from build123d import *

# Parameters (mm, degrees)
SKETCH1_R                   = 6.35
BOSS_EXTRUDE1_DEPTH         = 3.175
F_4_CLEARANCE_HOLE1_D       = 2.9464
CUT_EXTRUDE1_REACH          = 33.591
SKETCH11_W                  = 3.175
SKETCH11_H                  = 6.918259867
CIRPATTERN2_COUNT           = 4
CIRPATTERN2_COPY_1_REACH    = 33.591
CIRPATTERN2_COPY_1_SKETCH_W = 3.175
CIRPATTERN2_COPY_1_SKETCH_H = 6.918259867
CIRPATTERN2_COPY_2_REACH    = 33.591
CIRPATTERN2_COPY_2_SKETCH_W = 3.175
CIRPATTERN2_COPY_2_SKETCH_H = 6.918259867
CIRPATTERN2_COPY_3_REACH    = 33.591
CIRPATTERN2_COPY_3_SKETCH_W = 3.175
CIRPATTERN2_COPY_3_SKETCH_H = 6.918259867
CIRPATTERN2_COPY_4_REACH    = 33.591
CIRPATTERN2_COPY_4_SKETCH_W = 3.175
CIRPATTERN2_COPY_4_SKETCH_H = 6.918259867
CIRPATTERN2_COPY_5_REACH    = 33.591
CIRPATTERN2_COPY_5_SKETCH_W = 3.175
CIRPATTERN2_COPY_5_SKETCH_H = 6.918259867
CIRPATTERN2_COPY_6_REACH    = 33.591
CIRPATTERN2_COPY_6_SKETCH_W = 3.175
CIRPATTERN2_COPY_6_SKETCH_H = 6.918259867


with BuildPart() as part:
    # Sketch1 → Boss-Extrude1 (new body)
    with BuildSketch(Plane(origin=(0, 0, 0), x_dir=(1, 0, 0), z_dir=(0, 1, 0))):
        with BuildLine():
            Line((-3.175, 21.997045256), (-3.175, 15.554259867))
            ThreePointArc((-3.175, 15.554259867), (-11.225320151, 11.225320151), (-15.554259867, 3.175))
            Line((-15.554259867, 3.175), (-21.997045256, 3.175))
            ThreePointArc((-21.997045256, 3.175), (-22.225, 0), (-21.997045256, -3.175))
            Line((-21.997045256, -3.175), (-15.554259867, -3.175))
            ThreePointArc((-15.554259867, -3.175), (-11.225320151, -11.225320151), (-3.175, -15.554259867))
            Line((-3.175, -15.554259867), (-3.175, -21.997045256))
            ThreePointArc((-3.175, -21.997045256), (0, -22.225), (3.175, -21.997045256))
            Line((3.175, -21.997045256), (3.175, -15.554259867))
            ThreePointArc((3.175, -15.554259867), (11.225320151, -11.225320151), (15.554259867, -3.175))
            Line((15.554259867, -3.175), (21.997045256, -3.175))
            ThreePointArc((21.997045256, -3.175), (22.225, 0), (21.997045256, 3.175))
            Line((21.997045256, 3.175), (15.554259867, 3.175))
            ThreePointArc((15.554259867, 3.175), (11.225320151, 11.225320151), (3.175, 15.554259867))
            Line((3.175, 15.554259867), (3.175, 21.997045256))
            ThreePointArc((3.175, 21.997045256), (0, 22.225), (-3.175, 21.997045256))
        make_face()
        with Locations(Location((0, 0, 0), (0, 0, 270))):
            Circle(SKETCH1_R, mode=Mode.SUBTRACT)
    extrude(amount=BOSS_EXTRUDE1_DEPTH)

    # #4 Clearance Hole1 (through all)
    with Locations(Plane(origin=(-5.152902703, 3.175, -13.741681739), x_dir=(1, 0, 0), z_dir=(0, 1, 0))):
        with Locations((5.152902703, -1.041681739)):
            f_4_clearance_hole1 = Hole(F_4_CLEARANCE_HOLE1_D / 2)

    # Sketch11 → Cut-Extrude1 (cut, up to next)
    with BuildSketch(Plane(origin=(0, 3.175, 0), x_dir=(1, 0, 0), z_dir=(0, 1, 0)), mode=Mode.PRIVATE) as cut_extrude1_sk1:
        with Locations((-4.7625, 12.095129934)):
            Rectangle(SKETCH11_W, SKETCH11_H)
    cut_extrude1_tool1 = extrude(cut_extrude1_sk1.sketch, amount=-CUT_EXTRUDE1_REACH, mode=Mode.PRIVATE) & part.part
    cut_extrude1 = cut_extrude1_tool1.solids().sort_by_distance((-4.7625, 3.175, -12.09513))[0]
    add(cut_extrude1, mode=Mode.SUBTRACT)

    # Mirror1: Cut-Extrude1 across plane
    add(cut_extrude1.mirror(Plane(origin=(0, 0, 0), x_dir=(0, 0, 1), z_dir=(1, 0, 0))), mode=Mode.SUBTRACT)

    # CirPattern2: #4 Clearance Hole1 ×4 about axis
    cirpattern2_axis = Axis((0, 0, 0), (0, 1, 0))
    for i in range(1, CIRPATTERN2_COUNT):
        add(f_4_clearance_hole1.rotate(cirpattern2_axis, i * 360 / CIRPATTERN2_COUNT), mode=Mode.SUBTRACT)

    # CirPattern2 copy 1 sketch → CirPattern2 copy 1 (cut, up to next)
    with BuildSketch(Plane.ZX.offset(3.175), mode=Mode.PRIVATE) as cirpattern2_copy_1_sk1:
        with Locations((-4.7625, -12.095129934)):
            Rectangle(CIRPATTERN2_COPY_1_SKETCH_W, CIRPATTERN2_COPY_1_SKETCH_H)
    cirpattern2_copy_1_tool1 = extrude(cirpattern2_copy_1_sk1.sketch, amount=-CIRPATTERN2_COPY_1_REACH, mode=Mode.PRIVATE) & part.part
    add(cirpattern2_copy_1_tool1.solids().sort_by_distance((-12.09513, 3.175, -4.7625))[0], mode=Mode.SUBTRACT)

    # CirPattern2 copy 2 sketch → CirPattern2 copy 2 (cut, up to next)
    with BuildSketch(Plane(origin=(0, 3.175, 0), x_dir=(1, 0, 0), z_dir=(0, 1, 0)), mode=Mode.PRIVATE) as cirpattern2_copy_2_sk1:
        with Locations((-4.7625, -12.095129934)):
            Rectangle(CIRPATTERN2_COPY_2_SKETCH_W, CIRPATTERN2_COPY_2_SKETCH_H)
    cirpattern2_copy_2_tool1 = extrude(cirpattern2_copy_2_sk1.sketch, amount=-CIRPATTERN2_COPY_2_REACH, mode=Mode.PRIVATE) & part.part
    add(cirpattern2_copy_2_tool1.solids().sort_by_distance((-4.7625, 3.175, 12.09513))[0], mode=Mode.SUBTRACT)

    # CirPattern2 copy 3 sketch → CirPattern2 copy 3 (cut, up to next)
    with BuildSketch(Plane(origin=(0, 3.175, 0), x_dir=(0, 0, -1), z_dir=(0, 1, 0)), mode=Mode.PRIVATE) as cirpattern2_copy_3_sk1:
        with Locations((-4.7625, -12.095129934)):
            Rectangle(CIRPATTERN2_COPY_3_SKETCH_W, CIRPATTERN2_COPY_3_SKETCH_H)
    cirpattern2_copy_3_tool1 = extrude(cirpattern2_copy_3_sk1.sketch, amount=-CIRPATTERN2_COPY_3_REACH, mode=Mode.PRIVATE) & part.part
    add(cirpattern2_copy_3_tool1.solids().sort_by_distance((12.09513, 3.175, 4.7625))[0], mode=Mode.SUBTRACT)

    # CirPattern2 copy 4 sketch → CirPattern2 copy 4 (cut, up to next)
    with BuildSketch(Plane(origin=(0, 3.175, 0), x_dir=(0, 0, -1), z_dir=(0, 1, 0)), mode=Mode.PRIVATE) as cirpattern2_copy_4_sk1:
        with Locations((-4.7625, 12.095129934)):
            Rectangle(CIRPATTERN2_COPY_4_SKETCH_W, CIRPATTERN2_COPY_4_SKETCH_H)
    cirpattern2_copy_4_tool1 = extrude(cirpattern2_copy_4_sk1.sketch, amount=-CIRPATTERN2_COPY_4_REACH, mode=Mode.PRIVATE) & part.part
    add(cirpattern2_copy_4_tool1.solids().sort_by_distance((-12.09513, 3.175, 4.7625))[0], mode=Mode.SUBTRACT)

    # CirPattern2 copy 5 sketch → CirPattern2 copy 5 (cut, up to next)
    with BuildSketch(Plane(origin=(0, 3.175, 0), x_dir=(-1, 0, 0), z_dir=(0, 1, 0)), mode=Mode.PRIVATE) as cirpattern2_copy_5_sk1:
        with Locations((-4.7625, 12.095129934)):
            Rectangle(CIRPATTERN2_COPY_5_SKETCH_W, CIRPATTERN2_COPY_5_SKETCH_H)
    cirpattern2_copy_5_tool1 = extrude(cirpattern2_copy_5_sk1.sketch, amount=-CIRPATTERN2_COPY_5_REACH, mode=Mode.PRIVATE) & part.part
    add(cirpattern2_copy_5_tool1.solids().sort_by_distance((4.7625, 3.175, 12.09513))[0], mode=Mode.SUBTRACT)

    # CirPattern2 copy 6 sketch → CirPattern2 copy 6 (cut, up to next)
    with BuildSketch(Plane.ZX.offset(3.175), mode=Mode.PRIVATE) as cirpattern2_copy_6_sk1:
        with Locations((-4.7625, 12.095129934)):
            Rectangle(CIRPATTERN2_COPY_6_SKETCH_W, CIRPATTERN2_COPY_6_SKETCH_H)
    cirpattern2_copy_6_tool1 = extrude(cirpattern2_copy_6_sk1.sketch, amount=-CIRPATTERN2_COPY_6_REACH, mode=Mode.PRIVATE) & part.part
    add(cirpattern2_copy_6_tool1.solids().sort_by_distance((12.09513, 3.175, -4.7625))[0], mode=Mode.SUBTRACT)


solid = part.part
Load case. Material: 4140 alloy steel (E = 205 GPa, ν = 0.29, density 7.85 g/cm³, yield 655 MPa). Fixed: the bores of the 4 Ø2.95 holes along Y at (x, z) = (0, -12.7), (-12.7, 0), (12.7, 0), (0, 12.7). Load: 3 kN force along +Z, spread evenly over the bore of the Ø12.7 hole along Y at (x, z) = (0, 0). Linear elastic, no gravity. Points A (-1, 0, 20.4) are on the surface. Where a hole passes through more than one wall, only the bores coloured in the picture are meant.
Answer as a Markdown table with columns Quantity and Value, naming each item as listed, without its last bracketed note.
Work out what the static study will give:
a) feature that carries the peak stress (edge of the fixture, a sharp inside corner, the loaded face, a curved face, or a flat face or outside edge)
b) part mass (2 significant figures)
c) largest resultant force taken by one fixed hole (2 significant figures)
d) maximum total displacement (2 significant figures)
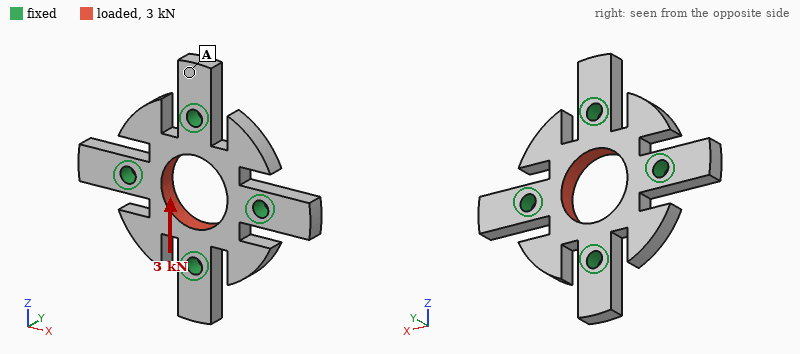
| Quantity | Value |
|---|---|
| feature that carries the peak stress | edge of the fixture |
| part mass | 16 g |
| largest resultant force taken by one fixed hole | 970 N |
| maximum total displacement | 5.3 µm |
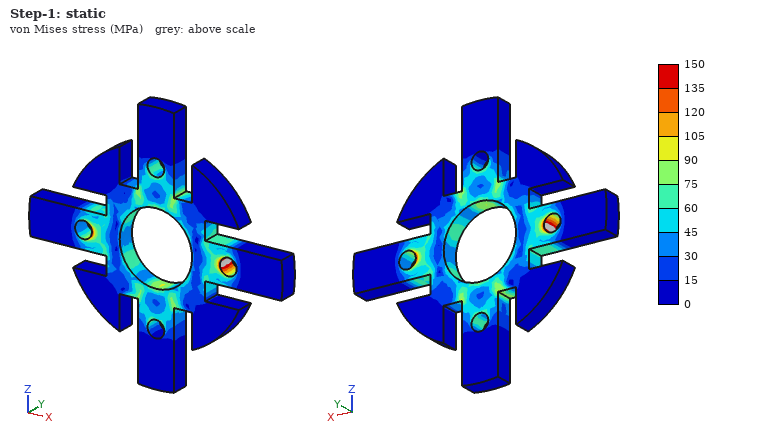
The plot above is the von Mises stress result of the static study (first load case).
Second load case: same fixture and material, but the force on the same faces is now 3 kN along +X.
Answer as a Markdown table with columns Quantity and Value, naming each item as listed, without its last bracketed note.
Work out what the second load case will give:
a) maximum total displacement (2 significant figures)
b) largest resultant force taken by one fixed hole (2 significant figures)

| Quantity | Value |
|---|---|
| maximum total displacement | 5.3 µm |
| largest resultant force taken by one fixed hole | 970 N |
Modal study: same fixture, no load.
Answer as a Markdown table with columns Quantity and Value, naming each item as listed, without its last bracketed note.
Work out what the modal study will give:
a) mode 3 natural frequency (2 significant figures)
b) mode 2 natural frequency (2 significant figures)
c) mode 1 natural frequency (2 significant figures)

| Quantity | Value |
|---|---|
| mode 3 natural frequency | 15 kHz |
| mode 2 natural frequency | 15 kHz |
| mode 1 natural frequency | 14 kHz |
